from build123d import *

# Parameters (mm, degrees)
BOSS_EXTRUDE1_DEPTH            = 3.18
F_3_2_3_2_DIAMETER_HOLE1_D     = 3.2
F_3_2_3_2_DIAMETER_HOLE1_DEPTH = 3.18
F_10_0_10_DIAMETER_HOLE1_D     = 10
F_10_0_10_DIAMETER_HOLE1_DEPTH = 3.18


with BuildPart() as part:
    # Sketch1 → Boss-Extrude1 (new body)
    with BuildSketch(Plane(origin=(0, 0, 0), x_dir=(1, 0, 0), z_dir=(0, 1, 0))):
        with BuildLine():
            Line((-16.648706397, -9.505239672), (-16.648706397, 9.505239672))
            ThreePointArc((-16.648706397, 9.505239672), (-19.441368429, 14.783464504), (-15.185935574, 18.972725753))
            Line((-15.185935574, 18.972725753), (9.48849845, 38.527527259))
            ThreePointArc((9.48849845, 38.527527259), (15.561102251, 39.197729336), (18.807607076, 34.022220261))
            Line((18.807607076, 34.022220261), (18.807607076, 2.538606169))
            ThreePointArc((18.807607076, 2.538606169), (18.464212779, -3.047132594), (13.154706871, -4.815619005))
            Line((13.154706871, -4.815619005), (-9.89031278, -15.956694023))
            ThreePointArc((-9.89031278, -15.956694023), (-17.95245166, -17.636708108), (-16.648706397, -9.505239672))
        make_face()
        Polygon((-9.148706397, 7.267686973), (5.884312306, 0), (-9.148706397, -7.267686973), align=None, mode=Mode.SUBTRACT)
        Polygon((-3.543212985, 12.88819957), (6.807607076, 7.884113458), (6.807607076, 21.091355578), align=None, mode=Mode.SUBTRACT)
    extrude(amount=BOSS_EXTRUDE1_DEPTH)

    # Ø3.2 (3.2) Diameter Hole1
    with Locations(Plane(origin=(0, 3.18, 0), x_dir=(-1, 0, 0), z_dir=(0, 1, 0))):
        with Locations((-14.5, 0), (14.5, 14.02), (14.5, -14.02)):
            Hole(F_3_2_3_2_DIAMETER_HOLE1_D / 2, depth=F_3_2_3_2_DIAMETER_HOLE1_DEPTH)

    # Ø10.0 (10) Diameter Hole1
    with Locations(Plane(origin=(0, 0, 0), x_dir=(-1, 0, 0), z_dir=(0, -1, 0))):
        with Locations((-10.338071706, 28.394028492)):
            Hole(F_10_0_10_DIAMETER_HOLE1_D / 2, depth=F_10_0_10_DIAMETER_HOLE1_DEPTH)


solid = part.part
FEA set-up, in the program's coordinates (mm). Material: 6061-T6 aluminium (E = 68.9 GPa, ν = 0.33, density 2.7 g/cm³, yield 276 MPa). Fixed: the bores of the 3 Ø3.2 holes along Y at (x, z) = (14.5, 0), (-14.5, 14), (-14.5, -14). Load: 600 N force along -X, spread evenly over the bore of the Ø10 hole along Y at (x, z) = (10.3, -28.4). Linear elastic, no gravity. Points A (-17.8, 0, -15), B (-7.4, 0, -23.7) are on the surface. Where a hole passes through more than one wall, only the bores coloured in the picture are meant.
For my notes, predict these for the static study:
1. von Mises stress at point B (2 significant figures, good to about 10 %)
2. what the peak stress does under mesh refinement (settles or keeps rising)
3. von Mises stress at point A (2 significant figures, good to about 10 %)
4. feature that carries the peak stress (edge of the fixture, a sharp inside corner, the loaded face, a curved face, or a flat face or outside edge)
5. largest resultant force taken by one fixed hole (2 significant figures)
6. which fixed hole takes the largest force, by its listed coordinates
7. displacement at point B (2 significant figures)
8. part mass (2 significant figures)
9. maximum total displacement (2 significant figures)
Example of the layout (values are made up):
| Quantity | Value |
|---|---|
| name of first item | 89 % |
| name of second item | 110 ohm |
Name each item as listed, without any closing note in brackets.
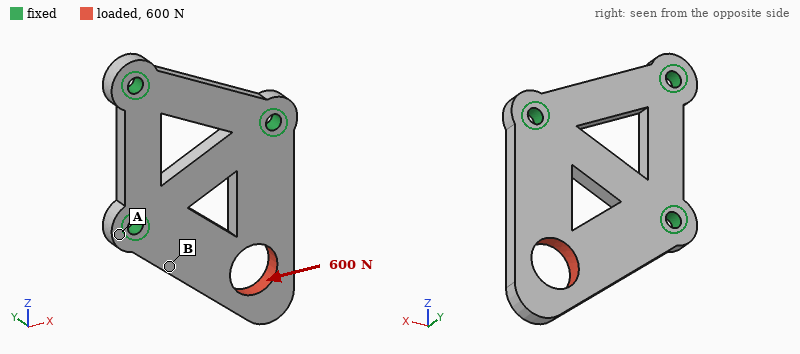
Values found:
| Quantity | Value |
|---|---|
| von Mises stress at point B | 21 MPa |
| what the peak stress does under mesh refinement | keeps rising |
| von Mises stress at point A | 8.4 MPa |
| feature that carries the peak stress | a sharp inside corner |
| largest resultant force taken by one fixed hole | 590 N |
| which fixed hole takes the largest force, by its listed coordinates | (-14.5, -14) |
| displacement at point B | 5.3 µm |
| part mass | 11 g |
| maximum total displacement | 20 µm |
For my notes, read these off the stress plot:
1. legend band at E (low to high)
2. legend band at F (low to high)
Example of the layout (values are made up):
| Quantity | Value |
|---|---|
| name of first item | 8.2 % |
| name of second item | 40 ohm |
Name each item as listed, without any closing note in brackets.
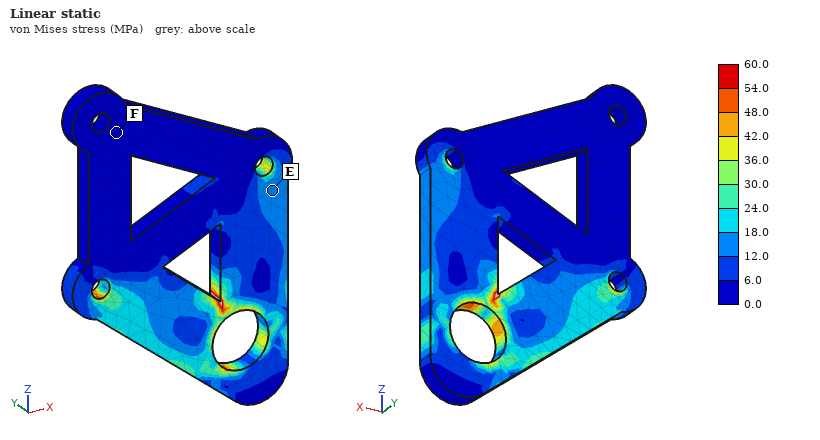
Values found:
| Quantity | Value |
|---|---|
| legend band at E | 12.0 to 18.0 MPa |
| legend band at F | 0.0 to 6.0 MPa |
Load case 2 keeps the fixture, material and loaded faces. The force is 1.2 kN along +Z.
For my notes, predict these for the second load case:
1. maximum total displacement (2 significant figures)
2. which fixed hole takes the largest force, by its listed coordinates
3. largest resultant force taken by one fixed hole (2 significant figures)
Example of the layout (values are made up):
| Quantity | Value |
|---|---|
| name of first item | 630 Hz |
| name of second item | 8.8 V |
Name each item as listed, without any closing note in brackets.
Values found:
| Quantity | Value |
|---|---|
| maximum total displacement | 22 µm |
| which fixed hole takes the largest force, by its listed coordinates | (14.5, 0) |
| largest resultant force taken by one fixed hole | 990 N |
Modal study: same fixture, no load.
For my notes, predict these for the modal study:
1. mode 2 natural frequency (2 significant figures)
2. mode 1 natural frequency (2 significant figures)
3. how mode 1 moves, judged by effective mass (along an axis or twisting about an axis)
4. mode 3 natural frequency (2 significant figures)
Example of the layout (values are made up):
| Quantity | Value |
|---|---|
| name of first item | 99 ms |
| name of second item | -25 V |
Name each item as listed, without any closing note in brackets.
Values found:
| Quantity | Value |
|---|---|
| mode 2 natural frequency | 10 kHz |
| mode 1 natural frequency | 2800 Hz |
| how mode 1 moves, judged by effective mass | along Y |
| mode 3 natural frequency | 11 kHz |
